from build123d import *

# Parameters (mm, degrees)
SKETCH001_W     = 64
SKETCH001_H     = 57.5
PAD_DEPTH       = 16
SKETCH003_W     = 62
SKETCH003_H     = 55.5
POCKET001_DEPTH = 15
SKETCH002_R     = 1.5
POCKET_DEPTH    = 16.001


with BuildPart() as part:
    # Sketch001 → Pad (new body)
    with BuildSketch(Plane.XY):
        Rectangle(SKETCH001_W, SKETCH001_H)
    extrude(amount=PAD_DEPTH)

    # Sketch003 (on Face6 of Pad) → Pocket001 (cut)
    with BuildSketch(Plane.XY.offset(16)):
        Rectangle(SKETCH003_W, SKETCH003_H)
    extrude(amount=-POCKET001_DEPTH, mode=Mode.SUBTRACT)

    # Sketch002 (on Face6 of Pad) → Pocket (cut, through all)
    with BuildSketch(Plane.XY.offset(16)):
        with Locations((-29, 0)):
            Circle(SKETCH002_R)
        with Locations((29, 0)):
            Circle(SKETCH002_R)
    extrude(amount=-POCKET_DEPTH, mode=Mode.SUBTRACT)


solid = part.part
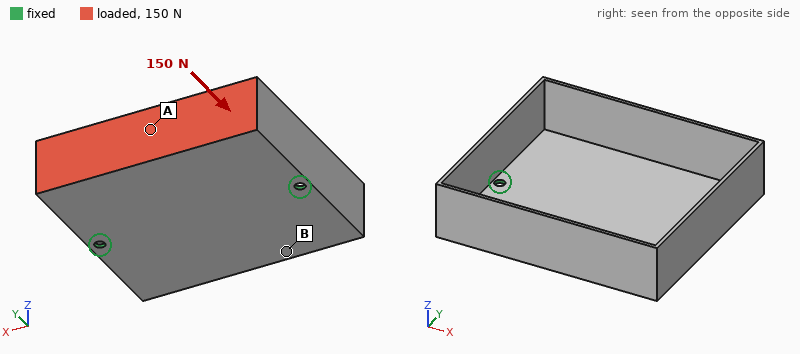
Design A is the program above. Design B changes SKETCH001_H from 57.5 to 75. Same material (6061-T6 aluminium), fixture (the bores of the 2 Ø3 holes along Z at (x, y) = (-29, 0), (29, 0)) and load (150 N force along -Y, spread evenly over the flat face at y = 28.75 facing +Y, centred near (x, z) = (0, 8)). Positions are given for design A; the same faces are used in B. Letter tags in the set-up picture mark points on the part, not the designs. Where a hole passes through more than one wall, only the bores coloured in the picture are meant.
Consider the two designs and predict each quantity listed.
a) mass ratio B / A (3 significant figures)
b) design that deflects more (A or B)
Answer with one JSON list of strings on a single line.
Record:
["3.47", "A"]
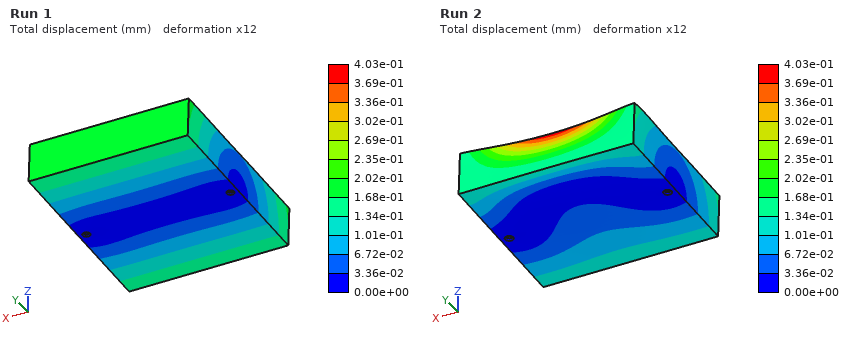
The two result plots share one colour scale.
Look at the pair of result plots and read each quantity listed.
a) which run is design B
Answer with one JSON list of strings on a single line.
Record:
["Run 1"]
